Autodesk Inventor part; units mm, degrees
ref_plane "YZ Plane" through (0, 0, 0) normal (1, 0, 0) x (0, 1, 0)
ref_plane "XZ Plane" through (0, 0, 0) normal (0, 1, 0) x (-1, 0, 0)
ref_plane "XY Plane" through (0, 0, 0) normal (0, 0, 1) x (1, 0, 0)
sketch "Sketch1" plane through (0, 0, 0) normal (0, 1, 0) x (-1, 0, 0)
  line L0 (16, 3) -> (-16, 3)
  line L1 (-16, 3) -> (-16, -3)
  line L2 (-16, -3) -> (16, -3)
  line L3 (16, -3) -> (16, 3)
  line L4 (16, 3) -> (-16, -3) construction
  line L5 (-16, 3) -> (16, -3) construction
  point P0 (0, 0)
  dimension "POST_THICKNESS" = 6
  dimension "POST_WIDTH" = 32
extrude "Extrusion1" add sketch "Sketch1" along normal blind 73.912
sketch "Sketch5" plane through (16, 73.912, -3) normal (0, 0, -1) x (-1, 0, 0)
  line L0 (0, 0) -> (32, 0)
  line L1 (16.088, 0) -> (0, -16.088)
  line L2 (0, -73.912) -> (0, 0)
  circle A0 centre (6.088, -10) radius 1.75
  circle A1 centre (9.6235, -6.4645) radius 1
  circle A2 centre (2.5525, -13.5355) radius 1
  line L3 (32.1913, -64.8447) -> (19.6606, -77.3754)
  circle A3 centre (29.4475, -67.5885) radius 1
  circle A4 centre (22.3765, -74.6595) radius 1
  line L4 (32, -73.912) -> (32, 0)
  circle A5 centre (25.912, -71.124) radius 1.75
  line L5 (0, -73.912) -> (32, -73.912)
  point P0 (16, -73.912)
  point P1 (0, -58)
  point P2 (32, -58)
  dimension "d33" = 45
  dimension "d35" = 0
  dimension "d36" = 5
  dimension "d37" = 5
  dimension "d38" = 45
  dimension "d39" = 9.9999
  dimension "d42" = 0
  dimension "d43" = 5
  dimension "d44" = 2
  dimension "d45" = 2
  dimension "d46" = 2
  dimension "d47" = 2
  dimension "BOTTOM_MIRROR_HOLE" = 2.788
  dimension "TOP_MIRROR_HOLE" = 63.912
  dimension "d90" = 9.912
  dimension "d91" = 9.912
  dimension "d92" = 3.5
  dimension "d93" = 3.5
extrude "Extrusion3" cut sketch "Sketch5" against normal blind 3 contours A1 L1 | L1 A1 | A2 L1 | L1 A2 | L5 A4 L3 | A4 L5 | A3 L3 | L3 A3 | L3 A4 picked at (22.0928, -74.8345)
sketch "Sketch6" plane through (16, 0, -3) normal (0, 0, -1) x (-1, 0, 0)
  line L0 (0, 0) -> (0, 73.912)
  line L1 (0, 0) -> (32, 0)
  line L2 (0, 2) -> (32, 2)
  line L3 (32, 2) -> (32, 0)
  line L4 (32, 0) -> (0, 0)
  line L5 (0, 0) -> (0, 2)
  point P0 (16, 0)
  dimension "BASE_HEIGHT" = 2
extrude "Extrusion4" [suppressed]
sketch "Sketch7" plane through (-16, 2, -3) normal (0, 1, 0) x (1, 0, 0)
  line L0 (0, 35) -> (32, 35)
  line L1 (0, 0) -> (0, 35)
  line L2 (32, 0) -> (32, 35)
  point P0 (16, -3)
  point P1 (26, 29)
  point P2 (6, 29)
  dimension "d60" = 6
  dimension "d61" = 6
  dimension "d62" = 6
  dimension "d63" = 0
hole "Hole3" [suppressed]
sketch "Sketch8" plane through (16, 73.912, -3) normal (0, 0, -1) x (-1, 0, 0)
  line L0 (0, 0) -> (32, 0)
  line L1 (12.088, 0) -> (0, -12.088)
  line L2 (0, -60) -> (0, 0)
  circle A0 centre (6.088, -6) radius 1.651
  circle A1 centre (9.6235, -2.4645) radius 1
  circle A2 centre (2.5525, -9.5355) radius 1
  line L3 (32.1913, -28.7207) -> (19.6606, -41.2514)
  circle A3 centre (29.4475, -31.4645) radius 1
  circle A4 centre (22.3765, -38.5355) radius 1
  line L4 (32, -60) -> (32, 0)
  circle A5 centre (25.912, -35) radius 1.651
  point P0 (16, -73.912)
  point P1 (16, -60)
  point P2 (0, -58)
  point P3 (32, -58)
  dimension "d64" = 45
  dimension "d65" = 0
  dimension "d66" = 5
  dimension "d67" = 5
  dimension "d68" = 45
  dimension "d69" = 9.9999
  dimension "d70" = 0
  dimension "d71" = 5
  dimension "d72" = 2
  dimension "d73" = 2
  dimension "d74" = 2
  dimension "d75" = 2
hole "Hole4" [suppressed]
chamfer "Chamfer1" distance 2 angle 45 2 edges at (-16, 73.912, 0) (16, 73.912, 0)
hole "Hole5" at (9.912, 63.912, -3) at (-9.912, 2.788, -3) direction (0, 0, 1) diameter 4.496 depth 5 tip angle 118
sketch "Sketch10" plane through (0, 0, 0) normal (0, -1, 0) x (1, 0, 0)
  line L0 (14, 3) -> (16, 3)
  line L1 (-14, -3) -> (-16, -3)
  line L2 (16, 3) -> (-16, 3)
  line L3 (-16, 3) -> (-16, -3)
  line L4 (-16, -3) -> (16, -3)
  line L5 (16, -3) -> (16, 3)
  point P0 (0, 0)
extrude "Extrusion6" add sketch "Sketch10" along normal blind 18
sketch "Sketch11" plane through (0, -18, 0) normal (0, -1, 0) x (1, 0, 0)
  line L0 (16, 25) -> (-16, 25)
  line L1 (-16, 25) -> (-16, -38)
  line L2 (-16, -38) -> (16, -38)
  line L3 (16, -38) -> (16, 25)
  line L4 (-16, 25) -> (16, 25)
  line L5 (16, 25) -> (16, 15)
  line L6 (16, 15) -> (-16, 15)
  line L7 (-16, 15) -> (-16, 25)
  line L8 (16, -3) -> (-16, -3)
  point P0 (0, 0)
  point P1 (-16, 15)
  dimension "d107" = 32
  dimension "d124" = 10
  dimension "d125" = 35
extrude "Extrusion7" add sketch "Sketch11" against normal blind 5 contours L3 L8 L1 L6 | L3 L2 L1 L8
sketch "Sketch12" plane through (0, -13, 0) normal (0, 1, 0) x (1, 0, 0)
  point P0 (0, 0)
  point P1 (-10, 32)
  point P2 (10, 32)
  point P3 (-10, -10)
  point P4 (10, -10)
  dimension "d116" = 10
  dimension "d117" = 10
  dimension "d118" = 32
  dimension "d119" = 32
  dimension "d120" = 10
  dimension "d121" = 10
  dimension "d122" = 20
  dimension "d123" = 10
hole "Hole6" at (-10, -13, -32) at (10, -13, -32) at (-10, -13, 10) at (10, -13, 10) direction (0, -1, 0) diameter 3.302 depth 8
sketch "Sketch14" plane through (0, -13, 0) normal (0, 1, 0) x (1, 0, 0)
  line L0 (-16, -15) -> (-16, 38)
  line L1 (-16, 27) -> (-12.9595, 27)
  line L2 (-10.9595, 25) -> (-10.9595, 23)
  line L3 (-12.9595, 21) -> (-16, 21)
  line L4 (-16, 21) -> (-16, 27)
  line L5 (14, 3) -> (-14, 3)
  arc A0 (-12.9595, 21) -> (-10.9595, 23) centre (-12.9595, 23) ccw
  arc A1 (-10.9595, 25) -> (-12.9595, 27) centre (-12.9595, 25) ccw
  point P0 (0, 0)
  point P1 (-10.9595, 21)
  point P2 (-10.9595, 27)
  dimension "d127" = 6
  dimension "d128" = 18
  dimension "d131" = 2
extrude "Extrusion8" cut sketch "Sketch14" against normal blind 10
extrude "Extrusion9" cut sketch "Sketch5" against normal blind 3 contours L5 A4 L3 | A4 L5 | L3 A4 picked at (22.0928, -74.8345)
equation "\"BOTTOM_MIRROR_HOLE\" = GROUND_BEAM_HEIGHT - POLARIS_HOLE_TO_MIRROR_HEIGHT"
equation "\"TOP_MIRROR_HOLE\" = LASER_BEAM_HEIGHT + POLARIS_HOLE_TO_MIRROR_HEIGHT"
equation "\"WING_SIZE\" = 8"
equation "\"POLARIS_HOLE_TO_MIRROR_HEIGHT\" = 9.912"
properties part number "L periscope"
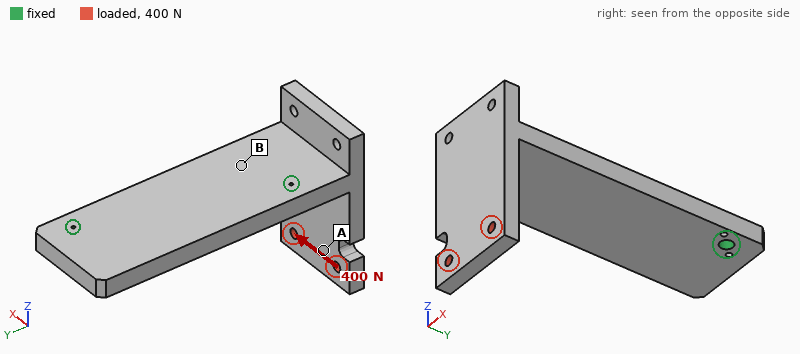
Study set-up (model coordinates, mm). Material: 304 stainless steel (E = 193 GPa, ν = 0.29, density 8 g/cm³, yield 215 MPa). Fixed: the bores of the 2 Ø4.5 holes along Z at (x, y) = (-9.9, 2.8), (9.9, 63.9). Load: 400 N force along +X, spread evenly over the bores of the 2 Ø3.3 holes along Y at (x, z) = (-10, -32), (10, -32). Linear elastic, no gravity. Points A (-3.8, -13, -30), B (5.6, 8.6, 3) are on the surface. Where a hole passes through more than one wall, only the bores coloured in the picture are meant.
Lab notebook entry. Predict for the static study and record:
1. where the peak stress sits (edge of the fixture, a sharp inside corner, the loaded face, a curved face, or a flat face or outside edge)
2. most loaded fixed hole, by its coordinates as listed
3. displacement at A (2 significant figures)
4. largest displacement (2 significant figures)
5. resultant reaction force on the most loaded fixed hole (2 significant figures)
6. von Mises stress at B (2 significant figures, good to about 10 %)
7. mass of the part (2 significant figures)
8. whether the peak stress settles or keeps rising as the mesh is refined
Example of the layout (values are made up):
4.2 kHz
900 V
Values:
edge of the fixture
(-9.9, 2.8)
58 µm
84 µm
480 N
30 MPa
200 g
keeps rising
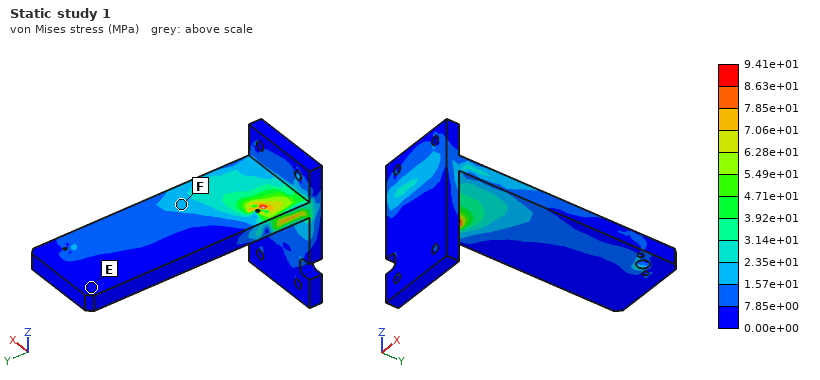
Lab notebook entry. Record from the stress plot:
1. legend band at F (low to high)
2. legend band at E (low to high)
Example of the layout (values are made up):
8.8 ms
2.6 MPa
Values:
1.57e+01 to 2.35e+01 MPa
0.00e+00 to 7.85e+00 MPa
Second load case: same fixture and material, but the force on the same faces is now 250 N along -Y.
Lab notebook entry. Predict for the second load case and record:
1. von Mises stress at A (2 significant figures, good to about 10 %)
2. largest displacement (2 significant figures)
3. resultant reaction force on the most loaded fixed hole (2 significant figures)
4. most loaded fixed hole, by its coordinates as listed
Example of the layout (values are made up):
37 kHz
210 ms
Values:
7.1 MPa
0.11 mm
210 N
(-9.9, 2.8)
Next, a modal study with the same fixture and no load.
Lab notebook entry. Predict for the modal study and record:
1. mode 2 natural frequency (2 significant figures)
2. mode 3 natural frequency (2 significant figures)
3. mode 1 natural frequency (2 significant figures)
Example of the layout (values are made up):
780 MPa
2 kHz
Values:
2300 Hz
4800 Hz
1700 Hz
